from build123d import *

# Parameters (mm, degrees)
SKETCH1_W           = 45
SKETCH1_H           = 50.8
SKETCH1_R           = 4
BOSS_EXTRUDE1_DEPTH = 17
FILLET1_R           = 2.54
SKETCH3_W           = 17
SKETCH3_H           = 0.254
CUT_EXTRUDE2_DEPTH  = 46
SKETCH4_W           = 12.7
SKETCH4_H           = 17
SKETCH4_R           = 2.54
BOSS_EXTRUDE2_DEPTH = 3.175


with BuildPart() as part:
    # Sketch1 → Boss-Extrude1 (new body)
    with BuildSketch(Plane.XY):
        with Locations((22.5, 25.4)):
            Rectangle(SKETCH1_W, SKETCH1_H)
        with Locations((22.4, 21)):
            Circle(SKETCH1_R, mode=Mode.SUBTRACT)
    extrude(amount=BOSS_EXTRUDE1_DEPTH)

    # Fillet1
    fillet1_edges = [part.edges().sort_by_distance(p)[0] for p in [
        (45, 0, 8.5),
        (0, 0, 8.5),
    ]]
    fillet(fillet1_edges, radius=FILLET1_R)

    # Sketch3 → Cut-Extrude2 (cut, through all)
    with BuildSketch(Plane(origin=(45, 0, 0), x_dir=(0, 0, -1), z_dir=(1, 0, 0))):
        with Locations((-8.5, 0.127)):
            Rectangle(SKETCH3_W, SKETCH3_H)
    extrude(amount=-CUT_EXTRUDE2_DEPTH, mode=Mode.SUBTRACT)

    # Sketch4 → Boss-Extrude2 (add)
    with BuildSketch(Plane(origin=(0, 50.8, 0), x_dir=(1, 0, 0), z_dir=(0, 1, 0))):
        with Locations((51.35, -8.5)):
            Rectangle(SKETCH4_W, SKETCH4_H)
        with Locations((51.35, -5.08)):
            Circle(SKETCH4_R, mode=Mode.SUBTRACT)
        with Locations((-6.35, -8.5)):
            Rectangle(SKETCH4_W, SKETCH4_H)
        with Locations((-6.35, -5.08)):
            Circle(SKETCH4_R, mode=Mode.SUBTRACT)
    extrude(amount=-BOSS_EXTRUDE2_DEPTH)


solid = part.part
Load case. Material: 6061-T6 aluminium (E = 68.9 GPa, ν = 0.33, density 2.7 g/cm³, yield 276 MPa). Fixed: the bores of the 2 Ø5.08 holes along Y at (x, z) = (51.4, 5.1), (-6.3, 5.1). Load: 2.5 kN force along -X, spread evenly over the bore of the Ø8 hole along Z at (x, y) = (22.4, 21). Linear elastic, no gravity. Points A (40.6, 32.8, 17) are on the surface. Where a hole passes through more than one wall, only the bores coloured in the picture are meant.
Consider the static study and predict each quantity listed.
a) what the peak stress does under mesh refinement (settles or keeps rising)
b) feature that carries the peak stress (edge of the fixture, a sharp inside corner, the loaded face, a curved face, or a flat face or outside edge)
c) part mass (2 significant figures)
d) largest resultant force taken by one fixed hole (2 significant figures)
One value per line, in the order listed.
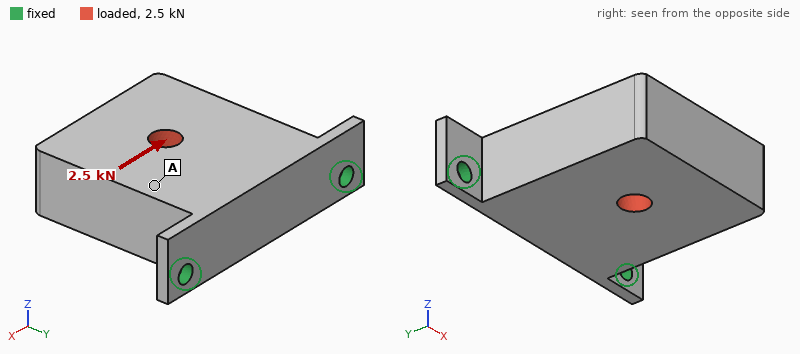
keeps rising
edge of the fixture
110 g
1.9 kN
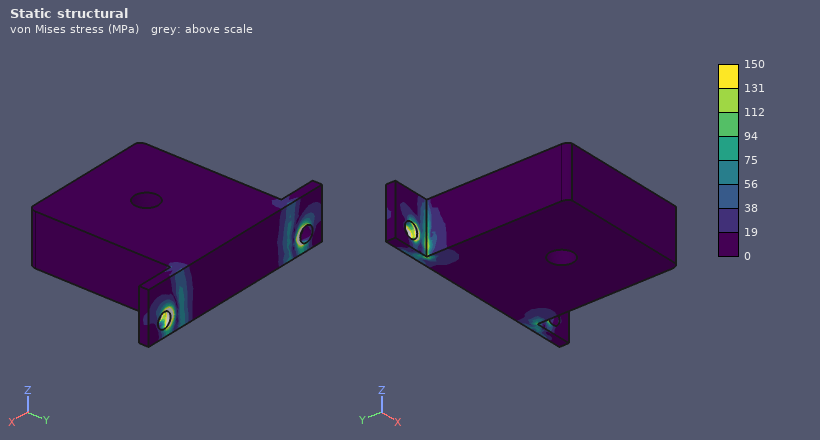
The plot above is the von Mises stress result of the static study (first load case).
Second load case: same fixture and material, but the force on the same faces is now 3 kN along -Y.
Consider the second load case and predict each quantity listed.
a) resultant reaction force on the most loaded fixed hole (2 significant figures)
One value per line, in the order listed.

1.7 kN
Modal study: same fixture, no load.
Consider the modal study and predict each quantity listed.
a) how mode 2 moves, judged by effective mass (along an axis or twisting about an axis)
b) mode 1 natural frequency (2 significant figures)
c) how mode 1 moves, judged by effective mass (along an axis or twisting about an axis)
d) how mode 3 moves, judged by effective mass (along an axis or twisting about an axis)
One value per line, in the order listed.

along X
760 Hz
along Z
along Y
